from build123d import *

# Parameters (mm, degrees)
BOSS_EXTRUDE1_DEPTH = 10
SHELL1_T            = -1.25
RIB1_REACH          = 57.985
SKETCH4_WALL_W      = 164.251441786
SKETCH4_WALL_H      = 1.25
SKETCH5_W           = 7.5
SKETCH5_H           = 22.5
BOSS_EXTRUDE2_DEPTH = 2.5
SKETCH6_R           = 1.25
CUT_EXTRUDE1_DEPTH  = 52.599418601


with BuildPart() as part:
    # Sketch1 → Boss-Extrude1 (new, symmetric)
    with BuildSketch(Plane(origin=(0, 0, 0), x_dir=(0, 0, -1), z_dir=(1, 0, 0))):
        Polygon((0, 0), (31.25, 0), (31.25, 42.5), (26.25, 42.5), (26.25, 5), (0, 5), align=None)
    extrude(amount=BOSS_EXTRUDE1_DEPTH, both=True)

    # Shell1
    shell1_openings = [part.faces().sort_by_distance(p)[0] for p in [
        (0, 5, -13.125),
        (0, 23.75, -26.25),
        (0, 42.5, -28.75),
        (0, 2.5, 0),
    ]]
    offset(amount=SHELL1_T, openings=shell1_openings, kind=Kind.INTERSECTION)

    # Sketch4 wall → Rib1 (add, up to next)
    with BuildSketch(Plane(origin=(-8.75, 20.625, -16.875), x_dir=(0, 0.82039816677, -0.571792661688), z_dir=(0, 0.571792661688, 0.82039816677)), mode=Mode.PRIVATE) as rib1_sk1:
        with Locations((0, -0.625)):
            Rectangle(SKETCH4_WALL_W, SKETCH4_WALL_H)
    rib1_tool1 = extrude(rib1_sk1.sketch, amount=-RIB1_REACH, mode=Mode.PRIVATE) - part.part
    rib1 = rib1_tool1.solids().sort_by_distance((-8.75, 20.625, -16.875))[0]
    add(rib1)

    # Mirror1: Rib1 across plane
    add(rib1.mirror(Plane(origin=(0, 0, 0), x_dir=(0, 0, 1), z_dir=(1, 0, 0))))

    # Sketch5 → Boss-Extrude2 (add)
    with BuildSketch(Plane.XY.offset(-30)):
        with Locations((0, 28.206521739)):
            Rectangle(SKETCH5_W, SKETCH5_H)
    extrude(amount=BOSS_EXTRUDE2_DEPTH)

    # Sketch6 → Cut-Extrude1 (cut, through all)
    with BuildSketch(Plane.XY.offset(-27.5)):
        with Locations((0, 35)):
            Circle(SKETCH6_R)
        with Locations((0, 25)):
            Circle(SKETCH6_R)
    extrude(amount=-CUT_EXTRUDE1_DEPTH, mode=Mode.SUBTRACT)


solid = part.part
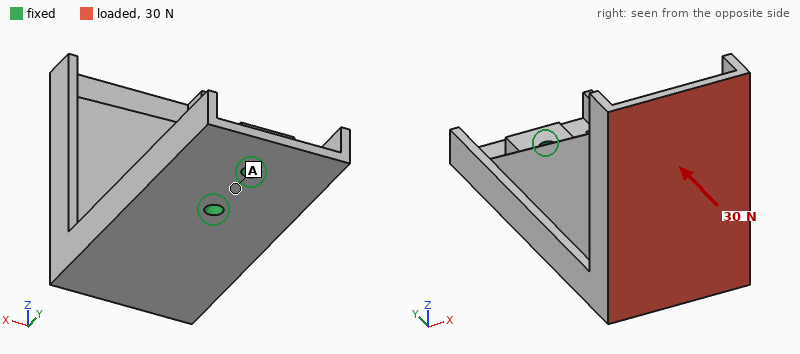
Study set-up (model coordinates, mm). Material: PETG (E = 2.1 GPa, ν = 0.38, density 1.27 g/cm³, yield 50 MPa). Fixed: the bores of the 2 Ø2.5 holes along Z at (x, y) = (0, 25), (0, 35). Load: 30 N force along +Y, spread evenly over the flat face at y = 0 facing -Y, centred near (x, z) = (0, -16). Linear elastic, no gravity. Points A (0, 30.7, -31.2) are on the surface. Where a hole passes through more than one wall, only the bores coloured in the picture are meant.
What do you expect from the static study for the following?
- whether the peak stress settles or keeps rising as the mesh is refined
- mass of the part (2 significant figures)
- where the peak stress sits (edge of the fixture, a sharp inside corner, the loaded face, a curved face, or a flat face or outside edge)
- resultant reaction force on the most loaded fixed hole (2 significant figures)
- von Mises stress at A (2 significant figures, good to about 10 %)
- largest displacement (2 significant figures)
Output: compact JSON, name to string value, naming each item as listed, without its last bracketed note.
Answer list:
{"whether the peak stress settles or keeps rising as the mesh is refined": "keeps rising", "mass of the part": "5.2 g", "where the peak stress sits": "edge of the fixture", "resultant reaction force on the most loaded fixed hole": "31 N", "von Mises stress at A": "1.1 MPa", "largest displacement": "0.58 mm"}
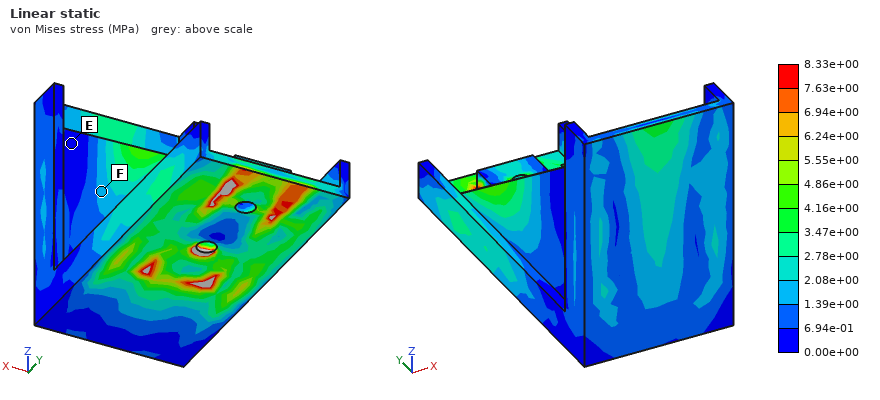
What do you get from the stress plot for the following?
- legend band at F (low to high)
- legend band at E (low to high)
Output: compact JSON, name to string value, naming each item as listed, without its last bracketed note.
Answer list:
{"legend band at F": "1.39e+00 to 2.08e+00 MPa", "legend band at E": "0.00e+00 to 6.94e-01 MPa"}
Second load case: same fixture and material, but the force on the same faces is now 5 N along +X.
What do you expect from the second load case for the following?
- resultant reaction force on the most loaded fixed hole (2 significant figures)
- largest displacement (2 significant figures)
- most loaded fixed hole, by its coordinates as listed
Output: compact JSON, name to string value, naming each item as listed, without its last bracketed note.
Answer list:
{"resultant reaction force on the most loaded fixed hole": "14 N", "largest displacement": "0.57 mm", "most loaded fixed hole, by its coordinates as listed": "(0, 25)"}
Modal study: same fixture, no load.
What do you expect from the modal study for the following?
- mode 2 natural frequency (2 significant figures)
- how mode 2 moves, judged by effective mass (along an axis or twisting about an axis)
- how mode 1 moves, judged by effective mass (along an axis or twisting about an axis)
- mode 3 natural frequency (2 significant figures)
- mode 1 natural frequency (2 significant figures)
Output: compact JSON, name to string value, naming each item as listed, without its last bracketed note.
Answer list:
{"mode 2 natural frequency": "650 Hz", "how mode 2 moves, judged by effective mass": "along Z", "how mode 1 moves, judged by effective mass": "along X", "mode 3 natural frequency": "1700 Hz", "mode 1 natural frequency": "380 Hz"}
